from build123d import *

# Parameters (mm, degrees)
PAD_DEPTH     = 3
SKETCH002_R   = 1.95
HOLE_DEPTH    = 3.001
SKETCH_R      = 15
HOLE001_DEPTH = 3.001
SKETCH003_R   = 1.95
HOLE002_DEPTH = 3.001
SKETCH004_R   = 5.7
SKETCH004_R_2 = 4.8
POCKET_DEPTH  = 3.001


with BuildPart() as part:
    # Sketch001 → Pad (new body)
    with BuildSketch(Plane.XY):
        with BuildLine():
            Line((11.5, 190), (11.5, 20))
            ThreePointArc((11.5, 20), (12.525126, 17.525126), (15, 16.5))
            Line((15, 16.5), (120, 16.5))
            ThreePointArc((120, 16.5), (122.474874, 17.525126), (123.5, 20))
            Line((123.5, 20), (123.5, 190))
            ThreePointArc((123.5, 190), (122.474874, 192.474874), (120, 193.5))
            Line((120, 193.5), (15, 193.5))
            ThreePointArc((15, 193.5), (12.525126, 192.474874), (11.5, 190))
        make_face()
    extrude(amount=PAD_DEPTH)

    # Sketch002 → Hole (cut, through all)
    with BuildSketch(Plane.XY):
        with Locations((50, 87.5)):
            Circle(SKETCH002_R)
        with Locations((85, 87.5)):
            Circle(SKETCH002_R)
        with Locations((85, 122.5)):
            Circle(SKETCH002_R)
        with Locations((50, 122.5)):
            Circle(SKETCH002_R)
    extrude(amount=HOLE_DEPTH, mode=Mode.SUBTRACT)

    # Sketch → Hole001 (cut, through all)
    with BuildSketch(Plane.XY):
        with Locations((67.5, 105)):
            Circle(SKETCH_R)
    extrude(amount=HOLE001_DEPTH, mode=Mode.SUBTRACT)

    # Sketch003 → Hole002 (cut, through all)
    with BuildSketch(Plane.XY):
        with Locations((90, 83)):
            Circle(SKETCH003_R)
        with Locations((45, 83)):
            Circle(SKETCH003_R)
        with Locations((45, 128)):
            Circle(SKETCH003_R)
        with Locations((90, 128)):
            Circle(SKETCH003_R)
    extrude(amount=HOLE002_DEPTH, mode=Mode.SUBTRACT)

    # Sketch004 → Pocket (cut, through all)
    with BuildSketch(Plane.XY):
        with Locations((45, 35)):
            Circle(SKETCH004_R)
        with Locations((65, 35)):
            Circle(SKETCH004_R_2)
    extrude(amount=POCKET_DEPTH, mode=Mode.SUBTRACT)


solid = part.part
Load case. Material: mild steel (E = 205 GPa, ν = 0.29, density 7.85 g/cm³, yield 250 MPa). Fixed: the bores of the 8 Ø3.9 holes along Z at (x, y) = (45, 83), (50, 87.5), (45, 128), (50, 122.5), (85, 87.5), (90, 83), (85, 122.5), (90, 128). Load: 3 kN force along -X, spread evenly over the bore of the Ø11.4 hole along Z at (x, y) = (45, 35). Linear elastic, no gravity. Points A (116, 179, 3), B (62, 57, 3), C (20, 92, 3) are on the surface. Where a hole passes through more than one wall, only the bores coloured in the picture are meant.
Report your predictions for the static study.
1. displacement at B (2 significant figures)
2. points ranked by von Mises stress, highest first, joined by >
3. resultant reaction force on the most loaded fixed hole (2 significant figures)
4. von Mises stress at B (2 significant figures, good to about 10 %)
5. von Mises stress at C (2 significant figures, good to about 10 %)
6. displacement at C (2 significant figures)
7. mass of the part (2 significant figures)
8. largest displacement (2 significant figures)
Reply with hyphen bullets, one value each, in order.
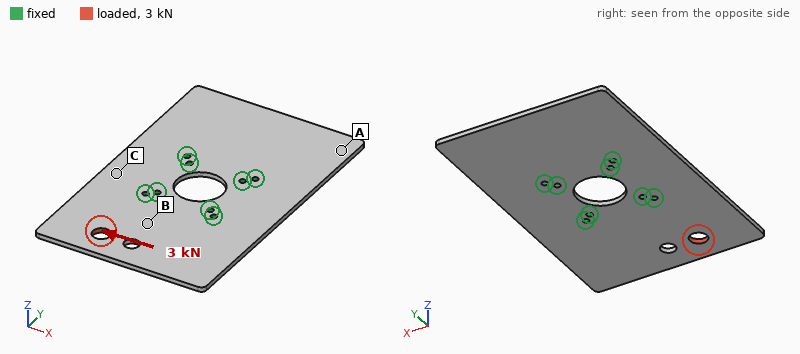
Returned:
- 6.6 µm
- B > C > A
- 1.8 kN
- 28 MPa
- 17 MPa
- 3.7 µm
- 440 g
- 20 µm
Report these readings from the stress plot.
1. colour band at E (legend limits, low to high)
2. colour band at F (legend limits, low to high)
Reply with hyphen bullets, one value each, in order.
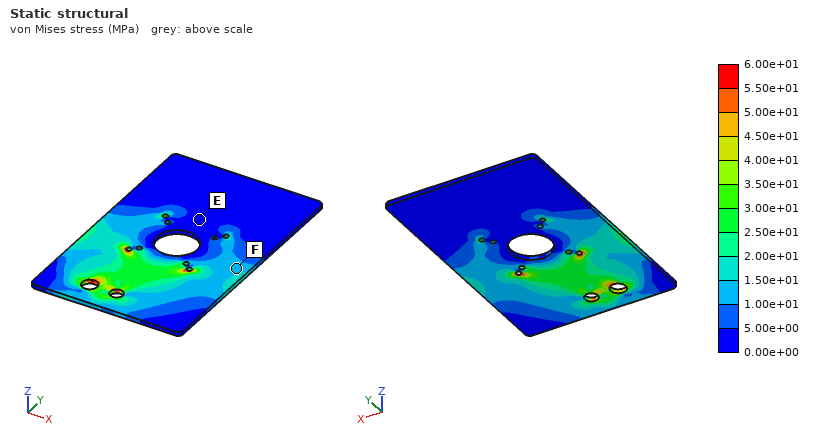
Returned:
- 0.00e+00 to 5.00e+00 MPa
- 1.00e+01 to 1.50e+01 MPa
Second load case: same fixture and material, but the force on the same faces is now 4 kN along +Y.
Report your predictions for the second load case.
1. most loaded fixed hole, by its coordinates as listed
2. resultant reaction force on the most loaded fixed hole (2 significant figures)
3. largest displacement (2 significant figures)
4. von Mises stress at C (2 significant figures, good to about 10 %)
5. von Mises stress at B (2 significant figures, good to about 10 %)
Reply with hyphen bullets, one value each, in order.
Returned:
- (45, 83)
- 1.8 kN
- 11 µm
- 14 MPa
- 20 MPa
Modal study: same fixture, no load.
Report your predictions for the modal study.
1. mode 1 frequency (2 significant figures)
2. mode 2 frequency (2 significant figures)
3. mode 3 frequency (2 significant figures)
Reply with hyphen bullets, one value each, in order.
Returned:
- 530 Hz
- 540 Hz
- 810 Hz
